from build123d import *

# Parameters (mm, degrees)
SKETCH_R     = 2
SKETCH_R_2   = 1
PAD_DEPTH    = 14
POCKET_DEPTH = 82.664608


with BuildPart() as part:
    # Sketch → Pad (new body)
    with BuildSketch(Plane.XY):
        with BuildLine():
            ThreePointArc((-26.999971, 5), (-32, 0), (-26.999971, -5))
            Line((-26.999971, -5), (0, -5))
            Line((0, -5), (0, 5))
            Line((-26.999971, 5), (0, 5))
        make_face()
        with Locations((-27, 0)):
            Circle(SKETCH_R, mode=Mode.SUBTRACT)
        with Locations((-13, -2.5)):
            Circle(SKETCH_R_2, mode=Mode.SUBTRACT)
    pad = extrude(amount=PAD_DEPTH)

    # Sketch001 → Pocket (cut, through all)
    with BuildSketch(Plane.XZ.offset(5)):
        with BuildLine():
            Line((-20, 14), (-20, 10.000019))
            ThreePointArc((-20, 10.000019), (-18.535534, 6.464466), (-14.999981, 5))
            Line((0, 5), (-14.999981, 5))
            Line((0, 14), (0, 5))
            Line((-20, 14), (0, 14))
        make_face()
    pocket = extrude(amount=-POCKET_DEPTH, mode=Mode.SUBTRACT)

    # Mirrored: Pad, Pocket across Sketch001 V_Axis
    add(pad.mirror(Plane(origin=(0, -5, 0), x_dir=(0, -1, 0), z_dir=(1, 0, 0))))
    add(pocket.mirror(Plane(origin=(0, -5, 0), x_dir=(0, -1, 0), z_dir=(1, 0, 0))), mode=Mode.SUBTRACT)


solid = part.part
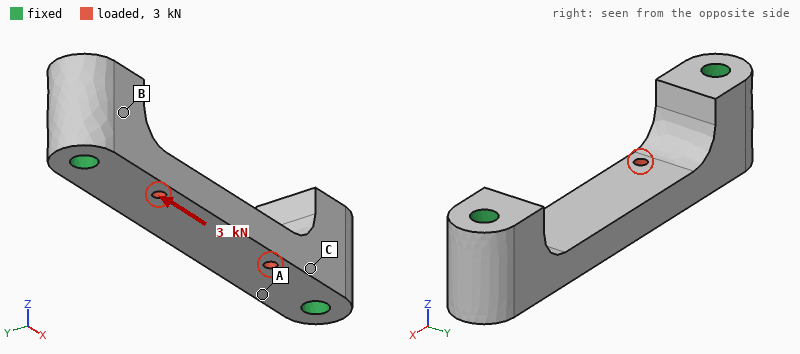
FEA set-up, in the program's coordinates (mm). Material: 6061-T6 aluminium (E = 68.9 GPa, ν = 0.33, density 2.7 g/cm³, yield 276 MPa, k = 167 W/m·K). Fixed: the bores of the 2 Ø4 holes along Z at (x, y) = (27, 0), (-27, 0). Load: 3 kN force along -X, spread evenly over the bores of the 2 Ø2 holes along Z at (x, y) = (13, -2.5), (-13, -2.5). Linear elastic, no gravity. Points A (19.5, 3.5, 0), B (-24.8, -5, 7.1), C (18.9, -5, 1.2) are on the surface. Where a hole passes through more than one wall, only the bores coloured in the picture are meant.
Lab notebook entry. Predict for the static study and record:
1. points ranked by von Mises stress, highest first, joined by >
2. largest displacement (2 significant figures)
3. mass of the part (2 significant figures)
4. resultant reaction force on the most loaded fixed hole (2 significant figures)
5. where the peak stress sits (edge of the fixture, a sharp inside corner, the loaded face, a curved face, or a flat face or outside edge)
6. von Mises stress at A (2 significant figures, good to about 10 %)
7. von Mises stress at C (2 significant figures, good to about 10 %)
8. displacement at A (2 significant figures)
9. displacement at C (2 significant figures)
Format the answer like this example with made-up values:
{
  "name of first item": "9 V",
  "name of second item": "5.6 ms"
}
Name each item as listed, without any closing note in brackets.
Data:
{
  "points ranked by von Mises stress, highest first, joined by >": "C > A > B",
  "largest displacement": "8.5 µm",
  "mass of the part": "13 g",
  "resultant reaction force on the most loaded fixed hole": "1.5 kN",
  "where the peak stress sits": "the loaded face",
  "von Mises stress at A": "20 MPa",
  "von Mises stress at C": "37 MPa",
  "displacement at A": "3.4 µm",
  "displacement at C": "4.2 µm"
}
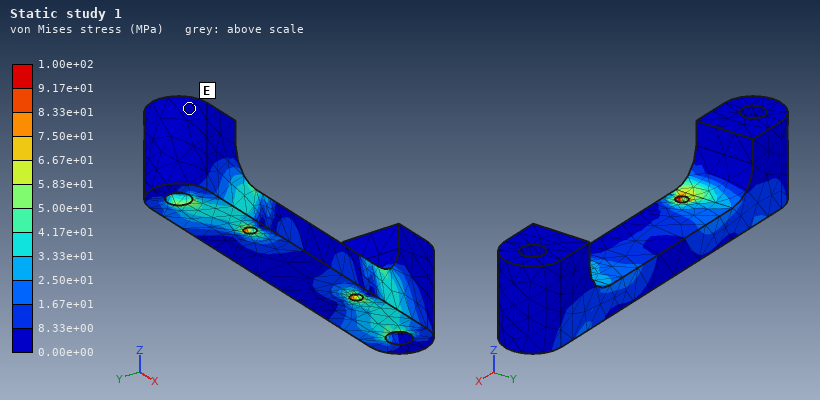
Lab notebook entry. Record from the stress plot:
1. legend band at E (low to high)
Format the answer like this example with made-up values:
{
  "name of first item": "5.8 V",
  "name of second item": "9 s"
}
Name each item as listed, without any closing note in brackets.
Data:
{
  "legend band at E": "0.00e+00 to 8.33e+00 MPa"
}
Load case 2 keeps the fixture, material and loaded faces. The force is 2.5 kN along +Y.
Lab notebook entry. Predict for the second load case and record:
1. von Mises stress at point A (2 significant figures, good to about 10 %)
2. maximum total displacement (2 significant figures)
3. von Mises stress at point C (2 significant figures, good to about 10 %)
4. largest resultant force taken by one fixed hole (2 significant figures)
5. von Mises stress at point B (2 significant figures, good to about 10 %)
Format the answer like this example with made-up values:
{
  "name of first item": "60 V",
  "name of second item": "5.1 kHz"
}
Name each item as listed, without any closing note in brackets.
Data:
{
  "von Mises stress at point A": "37 MPa",
  "maximum total displacement": "45 µm",
  "von Mises stress at point C": "35 MPa",
  "largest resultant force taken by one fixed hole": "1.3 kN",
  "von Mises stress at point B": "52 MPa"
}
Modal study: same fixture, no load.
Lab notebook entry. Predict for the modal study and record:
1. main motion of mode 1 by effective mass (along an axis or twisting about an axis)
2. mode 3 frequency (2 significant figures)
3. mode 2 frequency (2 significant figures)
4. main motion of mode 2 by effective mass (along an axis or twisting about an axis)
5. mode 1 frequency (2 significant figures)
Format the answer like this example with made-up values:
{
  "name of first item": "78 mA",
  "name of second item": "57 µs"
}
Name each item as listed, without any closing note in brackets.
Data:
{
  "main motion of mode 1 by effective mass": "along Z",
  "mode 3 frequency": "29 kHz",
  "mode 2 frequency": "16 kHz",
  "main motion of mode 2 by effective mass": "along Y",
  "mode 1 frequency": "14 kHz"
}
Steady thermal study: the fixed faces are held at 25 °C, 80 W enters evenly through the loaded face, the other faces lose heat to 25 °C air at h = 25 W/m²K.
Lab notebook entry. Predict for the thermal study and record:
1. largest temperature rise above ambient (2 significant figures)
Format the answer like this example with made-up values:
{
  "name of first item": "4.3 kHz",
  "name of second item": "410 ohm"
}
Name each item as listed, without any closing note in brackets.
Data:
{
  "largest temperature rise above ambient": "59 K"
}
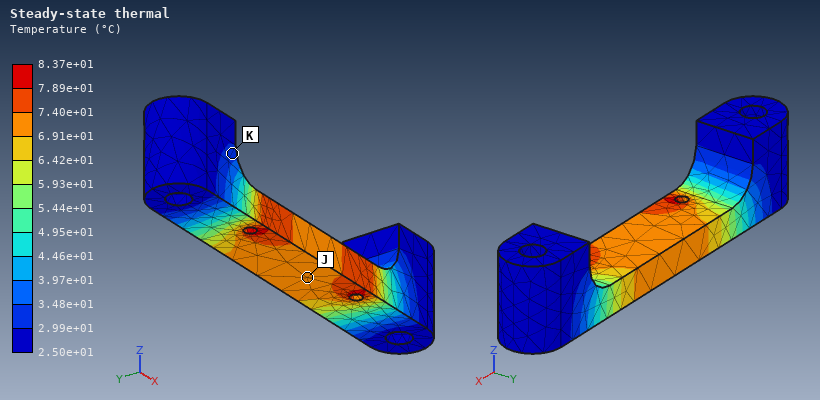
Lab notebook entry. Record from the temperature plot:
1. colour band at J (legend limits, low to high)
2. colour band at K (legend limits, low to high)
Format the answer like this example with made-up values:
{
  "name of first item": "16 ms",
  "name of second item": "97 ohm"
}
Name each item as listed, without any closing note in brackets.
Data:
{
  "colour band at J": "6.91e+01 to 7.40e+01 °C",
  "colour band at K": "2.99e+01 to 3.48e+01 °C"
}
